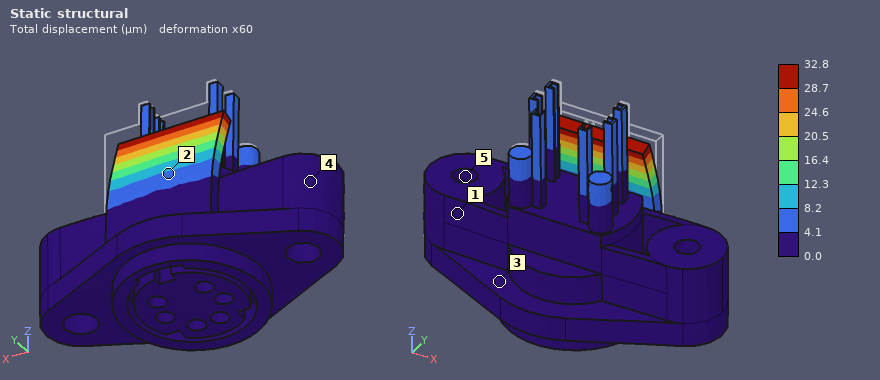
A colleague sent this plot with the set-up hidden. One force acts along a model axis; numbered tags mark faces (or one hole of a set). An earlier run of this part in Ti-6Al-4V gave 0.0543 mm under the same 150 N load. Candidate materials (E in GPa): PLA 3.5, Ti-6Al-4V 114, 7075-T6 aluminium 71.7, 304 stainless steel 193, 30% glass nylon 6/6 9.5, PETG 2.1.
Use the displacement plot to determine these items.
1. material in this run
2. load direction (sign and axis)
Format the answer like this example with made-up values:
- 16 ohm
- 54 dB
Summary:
- 304 stainless steel
- -Y
